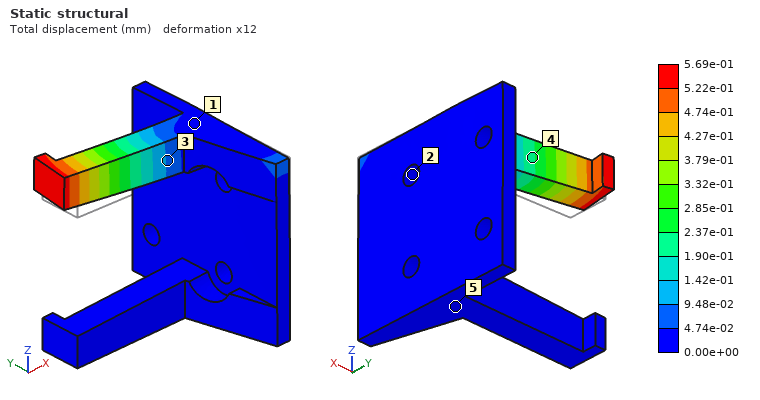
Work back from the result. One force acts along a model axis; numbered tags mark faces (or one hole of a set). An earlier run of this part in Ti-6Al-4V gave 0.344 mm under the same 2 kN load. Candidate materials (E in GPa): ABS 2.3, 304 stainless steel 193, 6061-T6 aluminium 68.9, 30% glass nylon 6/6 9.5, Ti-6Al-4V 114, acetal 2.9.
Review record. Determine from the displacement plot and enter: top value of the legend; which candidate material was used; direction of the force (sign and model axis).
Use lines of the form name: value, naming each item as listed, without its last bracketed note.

top value of the legend: 5.69e-01 mm
which candidate material was used: 6061-T6 aluminium
direction of the force: +Y
